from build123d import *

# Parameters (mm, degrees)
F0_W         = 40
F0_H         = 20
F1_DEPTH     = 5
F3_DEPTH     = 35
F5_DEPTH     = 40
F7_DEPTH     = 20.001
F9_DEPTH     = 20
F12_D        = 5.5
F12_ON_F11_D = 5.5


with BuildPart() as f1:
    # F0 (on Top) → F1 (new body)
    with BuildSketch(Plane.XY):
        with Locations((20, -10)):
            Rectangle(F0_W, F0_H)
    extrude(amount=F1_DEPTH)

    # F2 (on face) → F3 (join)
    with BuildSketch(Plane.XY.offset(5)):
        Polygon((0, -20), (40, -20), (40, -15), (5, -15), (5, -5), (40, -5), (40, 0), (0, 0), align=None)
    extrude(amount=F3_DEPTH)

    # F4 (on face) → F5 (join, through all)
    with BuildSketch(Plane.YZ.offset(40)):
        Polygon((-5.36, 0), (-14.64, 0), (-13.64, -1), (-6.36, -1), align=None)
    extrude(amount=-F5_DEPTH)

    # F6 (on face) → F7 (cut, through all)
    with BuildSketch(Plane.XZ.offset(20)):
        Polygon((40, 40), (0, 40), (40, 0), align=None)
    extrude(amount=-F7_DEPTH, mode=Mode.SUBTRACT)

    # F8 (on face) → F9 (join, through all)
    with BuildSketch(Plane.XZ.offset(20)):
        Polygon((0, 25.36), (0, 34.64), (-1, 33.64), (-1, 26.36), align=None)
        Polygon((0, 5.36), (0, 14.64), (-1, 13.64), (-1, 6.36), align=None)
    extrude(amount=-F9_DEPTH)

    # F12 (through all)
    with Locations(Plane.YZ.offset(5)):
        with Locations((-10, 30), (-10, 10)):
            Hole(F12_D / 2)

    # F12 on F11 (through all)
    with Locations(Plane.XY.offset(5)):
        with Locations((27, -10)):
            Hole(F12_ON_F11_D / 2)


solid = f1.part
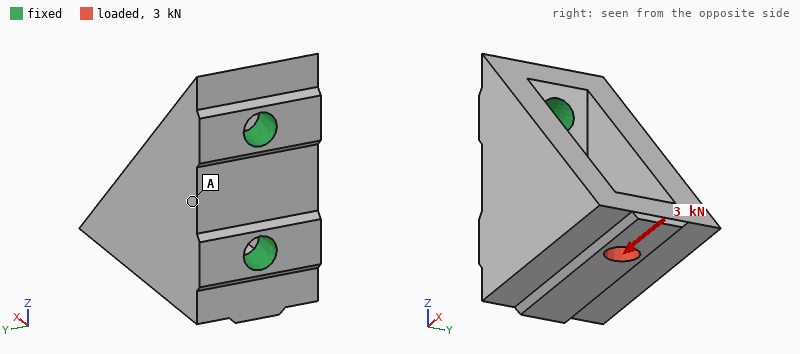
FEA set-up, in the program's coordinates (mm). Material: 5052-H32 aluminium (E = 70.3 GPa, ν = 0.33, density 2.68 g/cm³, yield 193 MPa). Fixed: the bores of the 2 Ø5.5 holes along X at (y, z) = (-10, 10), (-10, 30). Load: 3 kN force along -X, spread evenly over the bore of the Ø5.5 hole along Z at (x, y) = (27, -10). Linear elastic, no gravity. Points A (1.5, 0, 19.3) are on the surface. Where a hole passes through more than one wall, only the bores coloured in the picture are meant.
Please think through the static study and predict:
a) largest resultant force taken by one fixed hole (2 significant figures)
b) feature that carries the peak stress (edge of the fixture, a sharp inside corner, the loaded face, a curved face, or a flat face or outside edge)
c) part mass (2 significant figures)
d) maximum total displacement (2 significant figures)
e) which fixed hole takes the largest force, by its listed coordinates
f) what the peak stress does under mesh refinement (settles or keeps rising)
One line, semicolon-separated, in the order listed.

3.7 kN; edge of the fixture; 31 g; 45 µm; (-10, 10); keeps rising
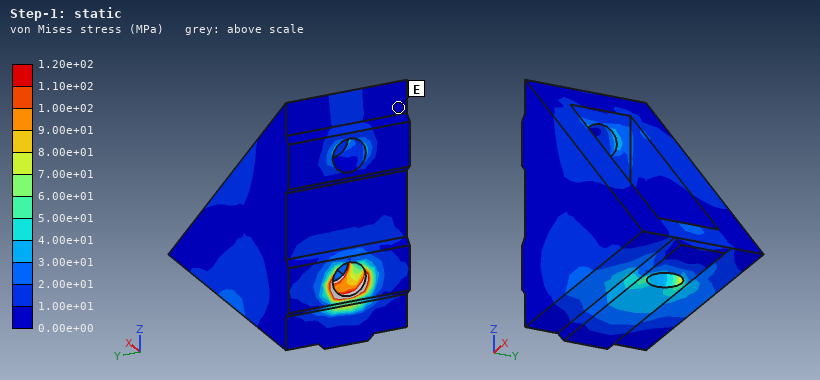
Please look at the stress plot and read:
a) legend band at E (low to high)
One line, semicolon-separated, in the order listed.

0.00e+00 to 1.00e+01 MPa
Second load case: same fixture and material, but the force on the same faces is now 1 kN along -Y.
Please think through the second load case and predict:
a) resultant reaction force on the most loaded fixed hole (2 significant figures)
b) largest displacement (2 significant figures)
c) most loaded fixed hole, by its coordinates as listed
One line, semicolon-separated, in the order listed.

1.2 kN; 91 µm; (-10, 10)
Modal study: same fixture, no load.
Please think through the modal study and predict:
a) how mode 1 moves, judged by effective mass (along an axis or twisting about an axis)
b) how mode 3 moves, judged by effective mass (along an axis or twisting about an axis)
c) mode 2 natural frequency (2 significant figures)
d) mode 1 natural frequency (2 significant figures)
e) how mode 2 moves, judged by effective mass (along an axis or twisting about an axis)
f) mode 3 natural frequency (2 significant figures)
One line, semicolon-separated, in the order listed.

along Y; along X; 11 kHz; 5900 Hz; along Z; 19 kHz
